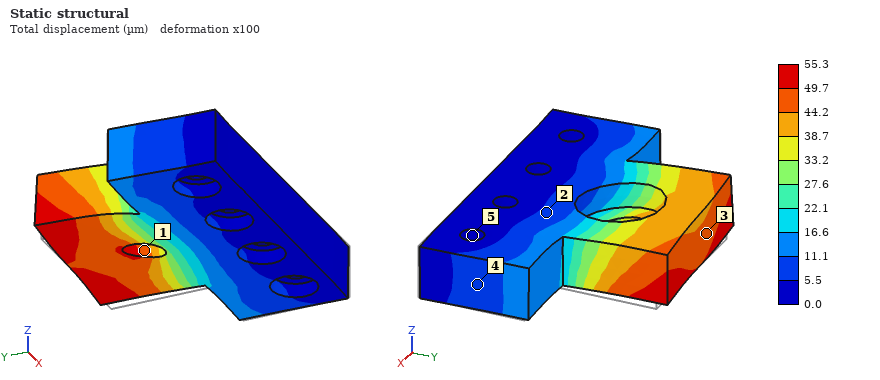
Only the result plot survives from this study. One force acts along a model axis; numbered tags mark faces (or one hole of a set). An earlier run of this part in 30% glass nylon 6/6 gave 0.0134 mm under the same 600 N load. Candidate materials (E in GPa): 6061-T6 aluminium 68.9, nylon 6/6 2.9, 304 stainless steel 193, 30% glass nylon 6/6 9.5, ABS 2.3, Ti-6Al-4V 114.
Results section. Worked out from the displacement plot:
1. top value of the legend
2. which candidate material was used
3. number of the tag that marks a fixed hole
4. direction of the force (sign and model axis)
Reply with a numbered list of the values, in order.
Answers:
1. 55.3 µm
2. ABS
3. 5
4. -X
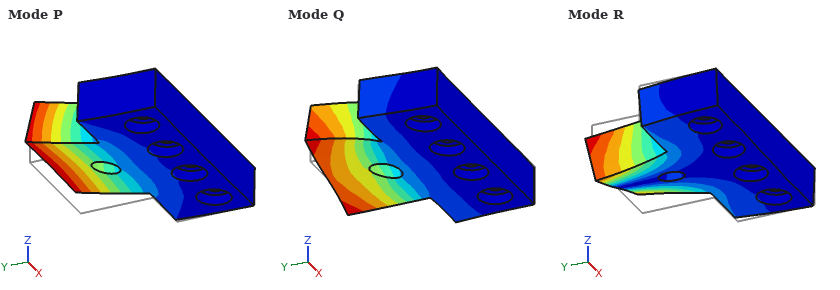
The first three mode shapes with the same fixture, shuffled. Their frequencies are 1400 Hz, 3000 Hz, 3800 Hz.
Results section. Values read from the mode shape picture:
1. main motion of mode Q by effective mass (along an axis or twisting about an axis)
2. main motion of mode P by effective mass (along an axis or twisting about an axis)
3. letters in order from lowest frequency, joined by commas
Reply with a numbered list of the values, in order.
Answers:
1. along X
2. along Z
3. P, R, Q
